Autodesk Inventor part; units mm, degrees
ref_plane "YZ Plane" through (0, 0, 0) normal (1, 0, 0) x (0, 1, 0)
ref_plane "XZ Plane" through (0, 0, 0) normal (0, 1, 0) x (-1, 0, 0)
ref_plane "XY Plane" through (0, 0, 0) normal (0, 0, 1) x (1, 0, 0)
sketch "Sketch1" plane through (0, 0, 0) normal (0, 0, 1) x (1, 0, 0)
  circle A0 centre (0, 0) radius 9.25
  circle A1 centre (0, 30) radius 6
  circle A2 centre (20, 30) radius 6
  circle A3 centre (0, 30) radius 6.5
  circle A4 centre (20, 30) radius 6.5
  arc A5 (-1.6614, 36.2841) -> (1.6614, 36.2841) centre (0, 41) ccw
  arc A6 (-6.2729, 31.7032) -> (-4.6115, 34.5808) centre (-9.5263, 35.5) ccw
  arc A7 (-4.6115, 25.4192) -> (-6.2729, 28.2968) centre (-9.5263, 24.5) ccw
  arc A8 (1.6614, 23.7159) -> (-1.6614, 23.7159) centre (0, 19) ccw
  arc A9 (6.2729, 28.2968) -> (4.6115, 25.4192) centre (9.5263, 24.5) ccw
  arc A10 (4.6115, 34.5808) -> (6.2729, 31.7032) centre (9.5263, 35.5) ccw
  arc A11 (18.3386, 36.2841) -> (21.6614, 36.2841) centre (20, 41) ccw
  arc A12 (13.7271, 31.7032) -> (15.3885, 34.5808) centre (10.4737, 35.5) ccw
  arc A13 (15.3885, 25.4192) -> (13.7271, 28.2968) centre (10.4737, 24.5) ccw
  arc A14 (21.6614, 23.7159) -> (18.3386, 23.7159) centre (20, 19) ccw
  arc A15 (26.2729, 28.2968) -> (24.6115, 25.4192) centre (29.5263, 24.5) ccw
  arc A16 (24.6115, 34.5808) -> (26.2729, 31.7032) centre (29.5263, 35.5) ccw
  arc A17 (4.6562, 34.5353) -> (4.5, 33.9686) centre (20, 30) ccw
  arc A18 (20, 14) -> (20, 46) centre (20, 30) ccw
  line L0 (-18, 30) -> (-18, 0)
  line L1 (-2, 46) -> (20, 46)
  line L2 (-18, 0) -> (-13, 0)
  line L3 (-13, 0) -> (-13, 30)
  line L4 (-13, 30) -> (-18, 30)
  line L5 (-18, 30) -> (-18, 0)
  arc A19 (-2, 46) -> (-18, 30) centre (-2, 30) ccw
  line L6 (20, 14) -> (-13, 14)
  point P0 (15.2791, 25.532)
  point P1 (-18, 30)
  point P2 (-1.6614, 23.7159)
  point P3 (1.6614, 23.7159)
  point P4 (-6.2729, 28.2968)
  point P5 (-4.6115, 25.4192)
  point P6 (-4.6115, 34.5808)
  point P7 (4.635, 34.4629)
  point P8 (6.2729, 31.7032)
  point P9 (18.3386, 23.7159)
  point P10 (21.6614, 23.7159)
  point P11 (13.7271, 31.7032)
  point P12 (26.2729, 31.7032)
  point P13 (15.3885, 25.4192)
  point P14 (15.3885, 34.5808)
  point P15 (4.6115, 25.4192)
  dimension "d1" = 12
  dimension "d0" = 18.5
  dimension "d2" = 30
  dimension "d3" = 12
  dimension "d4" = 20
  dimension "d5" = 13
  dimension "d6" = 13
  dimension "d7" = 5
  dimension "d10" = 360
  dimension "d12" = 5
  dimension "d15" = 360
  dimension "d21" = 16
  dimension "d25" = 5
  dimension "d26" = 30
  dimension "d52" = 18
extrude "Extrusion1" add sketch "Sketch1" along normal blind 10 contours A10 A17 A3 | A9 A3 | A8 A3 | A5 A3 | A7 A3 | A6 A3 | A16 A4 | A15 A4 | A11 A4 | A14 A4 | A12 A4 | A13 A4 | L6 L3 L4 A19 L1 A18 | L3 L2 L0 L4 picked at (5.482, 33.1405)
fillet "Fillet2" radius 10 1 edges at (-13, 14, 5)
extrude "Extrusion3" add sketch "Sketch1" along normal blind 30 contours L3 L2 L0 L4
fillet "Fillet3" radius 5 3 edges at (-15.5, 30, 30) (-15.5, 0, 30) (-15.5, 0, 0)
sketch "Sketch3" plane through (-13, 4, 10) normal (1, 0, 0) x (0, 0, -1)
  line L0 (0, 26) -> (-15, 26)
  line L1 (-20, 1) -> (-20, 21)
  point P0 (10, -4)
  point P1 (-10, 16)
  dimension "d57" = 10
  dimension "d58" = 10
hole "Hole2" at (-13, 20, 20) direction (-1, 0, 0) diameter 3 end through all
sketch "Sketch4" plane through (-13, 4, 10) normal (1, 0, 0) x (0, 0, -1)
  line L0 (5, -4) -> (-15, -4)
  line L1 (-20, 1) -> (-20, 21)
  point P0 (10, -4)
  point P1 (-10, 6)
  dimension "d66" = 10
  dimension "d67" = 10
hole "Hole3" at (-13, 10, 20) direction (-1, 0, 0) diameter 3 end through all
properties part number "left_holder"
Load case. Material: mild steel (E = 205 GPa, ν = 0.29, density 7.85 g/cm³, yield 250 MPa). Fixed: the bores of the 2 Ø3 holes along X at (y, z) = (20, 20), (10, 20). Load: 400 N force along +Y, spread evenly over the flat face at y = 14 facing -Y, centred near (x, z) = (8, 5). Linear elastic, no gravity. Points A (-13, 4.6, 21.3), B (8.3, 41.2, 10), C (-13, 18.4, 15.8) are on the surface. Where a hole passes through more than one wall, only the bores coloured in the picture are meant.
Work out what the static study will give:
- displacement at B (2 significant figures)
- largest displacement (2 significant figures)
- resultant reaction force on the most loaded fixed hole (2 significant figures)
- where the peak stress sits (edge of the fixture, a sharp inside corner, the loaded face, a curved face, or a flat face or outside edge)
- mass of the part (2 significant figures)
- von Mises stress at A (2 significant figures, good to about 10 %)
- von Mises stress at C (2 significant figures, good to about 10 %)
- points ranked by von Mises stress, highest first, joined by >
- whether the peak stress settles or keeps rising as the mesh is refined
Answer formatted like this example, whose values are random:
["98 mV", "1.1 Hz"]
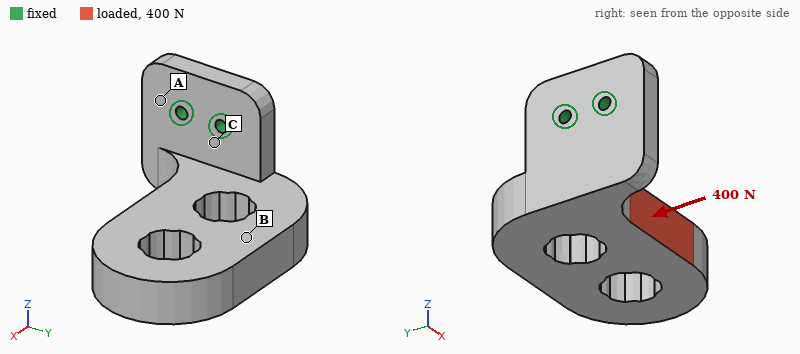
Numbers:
["30 µm", "48 µm", "790 N", "edge of the fixture", "130 g", "20 MPa", "51 MPa", "C > A > B", "keeps rising"]
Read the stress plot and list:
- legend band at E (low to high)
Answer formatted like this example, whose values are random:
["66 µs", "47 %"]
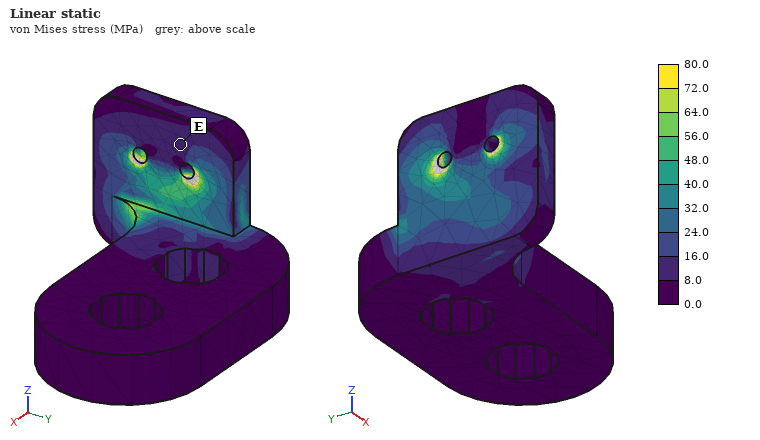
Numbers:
["8.0 to 16.0 MPa"]
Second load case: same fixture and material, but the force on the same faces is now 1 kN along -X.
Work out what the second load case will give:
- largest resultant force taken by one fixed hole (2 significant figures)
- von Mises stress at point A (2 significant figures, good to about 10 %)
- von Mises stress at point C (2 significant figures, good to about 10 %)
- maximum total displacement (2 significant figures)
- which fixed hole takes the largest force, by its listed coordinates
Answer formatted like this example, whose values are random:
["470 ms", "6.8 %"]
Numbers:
["560 N", "36 MPa", "99 MPa", "0.10 mm", "(10, 20)"]
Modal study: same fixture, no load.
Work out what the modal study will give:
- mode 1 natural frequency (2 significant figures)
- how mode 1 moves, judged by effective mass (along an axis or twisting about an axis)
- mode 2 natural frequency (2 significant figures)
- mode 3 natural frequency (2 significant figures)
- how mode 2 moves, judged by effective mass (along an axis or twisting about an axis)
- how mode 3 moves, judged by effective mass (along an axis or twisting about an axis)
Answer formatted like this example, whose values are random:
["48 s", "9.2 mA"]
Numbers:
["1100 Hz", "along Z", "1700 Hz", "5700 Hz", "along Y", "along X"]
